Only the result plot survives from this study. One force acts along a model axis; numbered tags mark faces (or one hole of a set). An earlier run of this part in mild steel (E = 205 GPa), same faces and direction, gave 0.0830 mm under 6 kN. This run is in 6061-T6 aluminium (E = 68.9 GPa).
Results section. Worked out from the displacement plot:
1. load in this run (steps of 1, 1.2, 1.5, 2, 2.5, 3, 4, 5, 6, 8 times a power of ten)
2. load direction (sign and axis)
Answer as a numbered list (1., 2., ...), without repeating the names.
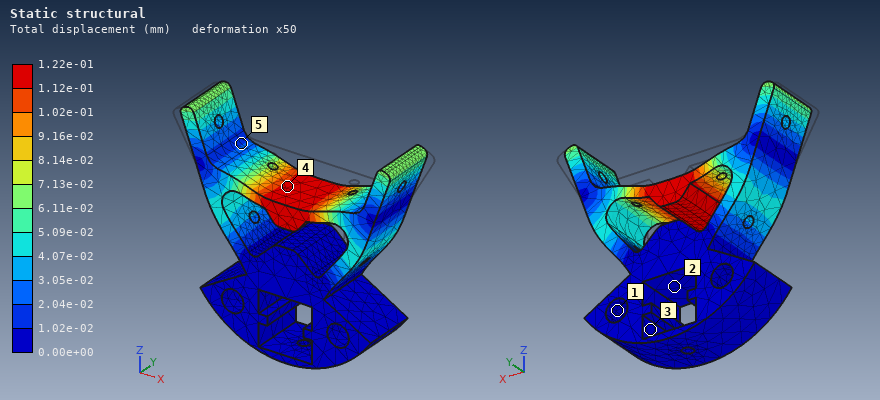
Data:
1. 3 kN
2. -Z
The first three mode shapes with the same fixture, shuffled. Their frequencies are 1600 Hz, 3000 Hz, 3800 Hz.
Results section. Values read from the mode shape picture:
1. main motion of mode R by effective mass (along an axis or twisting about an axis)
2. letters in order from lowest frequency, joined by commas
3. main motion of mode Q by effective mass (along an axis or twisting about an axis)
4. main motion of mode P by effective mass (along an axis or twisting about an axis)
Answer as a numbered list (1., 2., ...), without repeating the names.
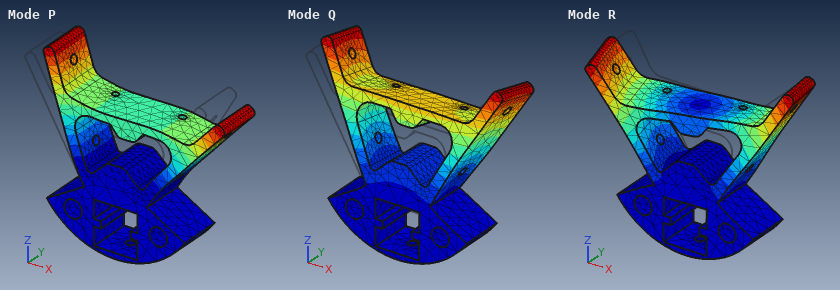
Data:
1. twisting about Z
2. P, Q, R
3. along Y
4. along X
